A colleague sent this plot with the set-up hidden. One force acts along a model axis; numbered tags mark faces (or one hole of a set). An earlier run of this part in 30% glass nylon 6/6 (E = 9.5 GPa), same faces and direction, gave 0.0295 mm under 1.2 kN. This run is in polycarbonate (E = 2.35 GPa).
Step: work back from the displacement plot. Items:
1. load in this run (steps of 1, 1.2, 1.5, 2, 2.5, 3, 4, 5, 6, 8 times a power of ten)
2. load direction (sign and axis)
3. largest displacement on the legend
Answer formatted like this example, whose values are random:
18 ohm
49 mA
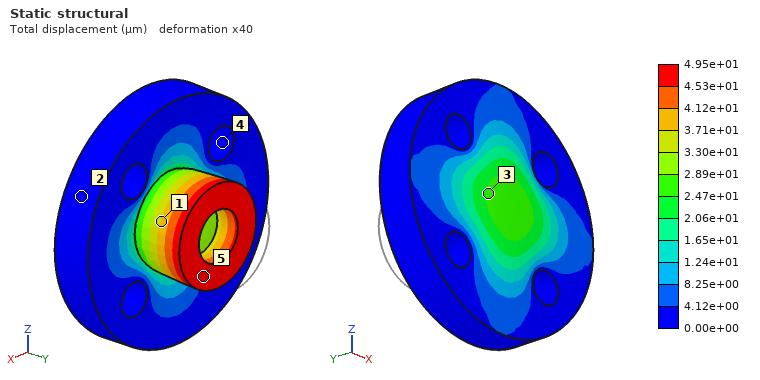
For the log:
500 N
-Y
4.95e+01 µm
